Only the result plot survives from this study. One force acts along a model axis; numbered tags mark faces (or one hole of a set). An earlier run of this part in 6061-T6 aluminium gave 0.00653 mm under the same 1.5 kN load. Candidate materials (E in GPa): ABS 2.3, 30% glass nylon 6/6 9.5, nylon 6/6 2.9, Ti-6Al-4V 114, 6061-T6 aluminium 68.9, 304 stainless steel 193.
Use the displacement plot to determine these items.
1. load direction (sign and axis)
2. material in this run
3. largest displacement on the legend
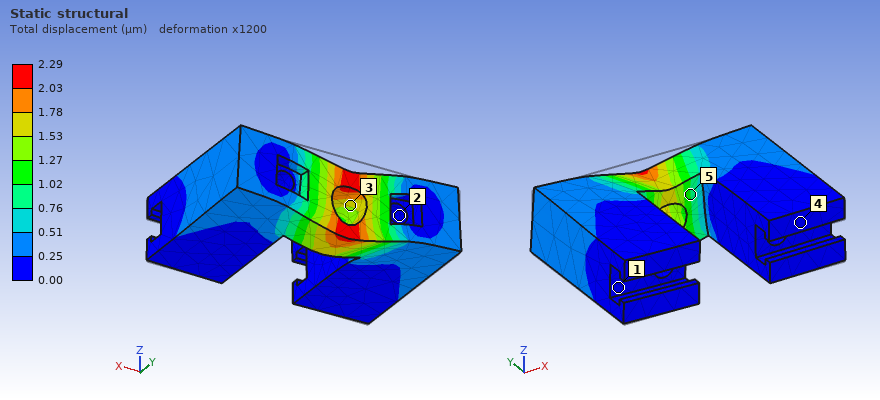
-Z
304 stainless steel
2.29 µm
